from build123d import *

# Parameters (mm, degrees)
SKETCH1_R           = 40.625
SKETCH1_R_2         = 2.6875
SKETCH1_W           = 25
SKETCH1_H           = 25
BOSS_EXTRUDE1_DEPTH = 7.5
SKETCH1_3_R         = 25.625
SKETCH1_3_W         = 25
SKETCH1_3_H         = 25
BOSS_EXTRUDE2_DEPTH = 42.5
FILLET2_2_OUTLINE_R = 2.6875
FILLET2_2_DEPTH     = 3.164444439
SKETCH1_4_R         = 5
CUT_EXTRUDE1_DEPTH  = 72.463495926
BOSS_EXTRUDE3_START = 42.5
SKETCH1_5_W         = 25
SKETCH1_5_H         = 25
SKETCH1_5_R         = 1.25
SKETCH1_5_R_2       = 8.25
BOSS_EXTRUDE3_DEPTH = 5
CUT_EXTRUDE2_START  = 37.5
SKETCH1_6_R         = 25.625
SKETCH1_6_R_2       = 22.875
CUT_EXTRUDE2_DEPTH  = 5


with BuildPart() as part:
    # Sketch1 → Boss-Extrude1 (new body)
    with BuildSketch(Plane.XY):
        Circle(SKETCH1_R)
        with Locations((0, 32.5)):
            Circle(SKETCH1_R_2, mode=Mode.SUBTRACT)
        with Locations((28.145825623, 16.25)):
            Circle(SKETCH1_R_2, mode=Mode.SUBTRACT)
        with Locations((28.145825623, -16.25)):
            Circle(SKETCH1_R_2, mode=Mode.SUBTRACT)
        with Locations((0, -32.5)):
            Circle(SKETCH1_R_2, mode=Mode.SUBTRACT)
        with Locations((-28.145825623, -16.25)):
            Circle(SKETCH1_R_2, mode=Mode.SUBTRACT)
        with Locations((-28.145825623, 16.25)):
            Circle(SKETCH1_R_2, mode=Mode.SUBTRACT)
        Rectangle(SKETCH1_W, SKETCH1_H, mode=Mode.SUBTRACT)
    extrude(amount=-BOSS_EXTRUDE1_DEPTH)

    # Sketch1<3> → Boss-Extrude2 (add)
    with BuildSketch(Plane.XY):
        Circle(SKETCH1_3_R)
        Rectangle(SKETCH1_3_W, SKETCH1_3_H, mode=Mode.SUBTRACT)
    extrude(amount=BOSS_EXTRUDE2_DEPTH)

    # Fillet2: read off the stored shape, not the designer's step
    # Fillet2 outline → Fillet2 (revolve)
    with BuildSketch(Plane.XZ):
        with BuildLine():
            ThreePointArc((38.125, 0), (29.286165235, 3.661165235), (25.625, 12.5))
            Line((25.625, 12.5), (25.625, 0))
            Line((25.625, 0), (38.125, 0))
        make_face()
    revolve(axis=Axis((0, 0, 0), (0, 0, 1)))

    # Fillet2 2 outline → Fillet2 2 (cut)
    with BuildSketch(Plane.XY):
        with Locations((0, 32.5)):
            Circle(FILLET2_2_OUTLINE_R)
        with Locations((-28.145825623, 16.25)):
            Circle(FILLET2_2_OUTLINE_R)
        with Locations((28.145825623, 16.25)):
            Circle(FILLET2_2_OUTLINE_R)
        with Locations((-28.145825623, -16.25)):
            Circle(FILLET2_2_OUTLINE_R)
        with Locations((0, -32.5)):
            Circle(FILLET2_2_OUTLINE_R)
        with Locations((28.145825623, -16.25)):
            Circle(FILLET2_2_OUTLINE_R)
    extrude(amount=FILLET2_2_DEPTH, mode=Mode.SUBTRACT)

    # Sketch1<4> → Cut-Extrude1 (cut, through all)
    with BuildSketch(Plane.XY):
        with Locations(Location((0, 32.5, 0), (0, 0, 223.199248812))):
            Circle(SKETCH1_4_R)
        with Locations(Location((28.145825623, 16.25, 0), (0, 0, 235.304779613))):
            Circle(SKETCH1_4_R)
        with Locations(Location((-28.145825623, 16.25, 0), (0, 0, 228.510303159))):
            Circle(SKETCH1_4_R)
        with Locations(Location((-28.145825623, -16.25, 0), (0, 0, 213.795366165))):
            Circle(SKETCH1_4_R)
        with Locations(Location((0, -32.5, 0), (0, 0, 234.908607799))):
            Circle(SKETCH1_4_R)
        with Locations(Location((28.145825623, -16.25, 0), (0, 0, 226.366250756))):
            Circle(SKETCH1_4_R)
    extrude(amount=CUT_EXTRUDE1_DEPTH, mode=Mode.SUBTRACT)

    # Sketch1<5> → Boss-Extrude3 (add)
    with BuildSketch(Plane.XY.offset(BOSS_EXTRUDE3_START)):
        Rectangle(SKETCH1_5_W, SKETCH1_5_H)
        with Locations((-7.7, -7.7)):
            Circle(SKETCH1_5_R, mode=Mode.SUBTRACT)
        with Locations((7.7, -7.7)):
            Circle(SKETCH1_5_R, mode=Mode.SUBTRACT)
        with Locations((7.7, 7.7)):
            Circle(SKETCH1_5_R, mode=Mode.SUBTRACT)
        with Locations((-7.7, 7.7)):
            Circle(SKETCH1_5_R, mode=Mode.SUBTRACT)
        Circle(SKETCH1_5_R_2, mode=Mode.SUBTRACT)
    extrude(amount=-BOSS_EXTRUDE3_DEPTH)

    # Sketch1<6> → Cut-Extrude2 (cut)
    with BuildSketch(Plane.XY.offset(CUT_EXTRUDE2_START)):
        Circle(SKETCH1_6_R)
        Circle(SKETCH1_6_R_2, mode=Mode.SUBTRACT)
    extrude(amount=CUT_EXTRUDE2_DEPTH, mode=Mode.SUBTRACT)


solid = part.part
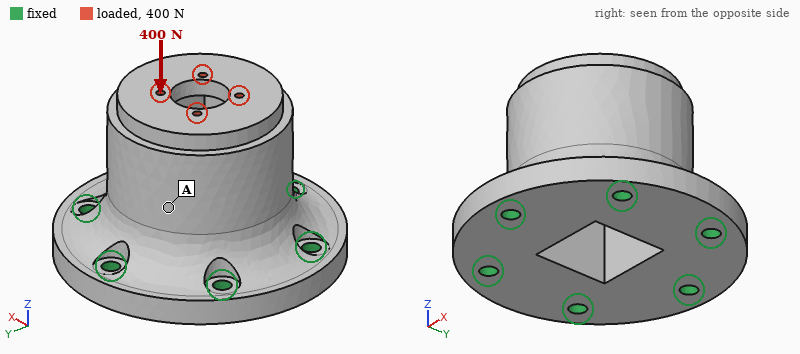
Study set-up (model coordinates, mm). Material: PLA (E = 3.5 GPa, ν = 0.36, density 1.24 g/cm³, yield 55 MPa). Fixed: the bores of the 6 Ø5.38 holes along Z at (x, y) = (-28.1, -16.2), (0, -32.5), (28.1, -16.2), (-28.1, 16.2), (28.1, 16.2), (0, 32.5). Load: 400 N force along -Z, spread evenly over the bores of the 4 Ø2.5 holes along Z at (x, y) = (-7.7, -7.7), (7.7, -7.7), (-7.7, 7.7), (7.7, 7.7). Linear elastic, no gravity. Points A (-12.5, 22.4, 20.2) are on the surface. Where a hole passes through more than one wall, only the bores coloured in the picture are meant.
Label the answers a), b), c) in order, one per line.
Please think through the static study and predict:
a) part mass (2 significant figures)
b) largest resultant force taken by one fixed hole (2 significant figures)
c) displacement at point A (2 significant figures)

a) 120 g
b) 75 N
c) 5.0 µm
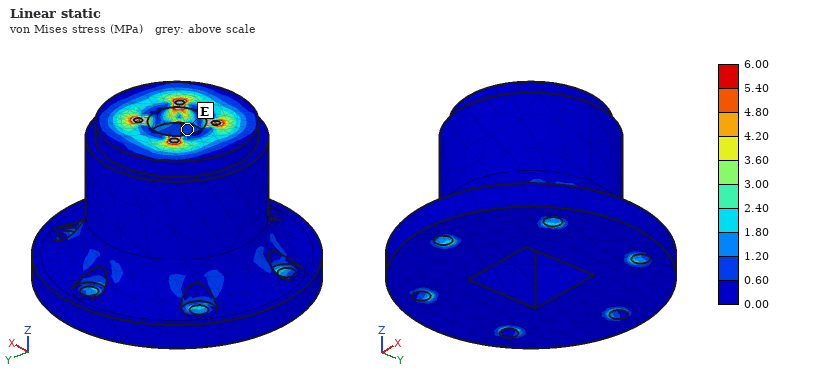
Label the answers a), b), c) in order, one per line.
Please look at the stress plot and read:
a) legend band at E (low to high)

a) 0.60 to 1.20 MPa
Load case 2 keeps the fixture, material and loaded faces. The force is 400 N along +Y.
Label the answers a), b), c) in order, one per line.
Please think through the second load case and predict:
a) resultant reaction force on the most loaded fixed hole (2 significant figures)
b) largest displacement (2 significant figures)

a) 210 N
b) 41 µm
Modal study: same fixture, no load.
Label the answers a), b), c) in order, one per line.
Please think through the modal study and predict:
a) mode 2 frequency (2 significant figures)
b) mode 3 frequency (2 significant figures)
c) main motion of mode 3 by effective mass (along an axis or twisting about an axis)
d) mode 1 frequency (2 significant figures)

a) 3200 Hz
b) 4800 Hz
c) along Z
d) 3200 Hz
